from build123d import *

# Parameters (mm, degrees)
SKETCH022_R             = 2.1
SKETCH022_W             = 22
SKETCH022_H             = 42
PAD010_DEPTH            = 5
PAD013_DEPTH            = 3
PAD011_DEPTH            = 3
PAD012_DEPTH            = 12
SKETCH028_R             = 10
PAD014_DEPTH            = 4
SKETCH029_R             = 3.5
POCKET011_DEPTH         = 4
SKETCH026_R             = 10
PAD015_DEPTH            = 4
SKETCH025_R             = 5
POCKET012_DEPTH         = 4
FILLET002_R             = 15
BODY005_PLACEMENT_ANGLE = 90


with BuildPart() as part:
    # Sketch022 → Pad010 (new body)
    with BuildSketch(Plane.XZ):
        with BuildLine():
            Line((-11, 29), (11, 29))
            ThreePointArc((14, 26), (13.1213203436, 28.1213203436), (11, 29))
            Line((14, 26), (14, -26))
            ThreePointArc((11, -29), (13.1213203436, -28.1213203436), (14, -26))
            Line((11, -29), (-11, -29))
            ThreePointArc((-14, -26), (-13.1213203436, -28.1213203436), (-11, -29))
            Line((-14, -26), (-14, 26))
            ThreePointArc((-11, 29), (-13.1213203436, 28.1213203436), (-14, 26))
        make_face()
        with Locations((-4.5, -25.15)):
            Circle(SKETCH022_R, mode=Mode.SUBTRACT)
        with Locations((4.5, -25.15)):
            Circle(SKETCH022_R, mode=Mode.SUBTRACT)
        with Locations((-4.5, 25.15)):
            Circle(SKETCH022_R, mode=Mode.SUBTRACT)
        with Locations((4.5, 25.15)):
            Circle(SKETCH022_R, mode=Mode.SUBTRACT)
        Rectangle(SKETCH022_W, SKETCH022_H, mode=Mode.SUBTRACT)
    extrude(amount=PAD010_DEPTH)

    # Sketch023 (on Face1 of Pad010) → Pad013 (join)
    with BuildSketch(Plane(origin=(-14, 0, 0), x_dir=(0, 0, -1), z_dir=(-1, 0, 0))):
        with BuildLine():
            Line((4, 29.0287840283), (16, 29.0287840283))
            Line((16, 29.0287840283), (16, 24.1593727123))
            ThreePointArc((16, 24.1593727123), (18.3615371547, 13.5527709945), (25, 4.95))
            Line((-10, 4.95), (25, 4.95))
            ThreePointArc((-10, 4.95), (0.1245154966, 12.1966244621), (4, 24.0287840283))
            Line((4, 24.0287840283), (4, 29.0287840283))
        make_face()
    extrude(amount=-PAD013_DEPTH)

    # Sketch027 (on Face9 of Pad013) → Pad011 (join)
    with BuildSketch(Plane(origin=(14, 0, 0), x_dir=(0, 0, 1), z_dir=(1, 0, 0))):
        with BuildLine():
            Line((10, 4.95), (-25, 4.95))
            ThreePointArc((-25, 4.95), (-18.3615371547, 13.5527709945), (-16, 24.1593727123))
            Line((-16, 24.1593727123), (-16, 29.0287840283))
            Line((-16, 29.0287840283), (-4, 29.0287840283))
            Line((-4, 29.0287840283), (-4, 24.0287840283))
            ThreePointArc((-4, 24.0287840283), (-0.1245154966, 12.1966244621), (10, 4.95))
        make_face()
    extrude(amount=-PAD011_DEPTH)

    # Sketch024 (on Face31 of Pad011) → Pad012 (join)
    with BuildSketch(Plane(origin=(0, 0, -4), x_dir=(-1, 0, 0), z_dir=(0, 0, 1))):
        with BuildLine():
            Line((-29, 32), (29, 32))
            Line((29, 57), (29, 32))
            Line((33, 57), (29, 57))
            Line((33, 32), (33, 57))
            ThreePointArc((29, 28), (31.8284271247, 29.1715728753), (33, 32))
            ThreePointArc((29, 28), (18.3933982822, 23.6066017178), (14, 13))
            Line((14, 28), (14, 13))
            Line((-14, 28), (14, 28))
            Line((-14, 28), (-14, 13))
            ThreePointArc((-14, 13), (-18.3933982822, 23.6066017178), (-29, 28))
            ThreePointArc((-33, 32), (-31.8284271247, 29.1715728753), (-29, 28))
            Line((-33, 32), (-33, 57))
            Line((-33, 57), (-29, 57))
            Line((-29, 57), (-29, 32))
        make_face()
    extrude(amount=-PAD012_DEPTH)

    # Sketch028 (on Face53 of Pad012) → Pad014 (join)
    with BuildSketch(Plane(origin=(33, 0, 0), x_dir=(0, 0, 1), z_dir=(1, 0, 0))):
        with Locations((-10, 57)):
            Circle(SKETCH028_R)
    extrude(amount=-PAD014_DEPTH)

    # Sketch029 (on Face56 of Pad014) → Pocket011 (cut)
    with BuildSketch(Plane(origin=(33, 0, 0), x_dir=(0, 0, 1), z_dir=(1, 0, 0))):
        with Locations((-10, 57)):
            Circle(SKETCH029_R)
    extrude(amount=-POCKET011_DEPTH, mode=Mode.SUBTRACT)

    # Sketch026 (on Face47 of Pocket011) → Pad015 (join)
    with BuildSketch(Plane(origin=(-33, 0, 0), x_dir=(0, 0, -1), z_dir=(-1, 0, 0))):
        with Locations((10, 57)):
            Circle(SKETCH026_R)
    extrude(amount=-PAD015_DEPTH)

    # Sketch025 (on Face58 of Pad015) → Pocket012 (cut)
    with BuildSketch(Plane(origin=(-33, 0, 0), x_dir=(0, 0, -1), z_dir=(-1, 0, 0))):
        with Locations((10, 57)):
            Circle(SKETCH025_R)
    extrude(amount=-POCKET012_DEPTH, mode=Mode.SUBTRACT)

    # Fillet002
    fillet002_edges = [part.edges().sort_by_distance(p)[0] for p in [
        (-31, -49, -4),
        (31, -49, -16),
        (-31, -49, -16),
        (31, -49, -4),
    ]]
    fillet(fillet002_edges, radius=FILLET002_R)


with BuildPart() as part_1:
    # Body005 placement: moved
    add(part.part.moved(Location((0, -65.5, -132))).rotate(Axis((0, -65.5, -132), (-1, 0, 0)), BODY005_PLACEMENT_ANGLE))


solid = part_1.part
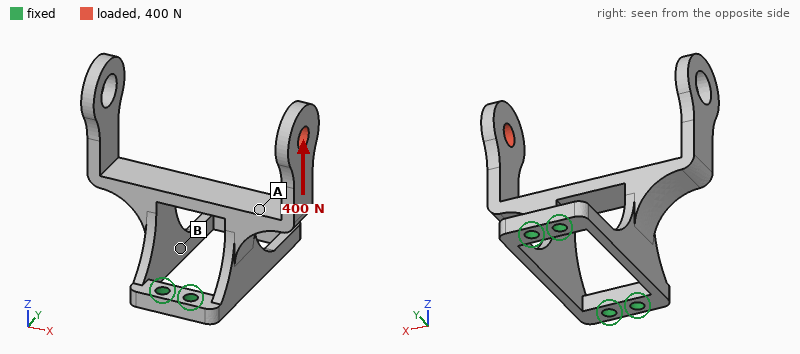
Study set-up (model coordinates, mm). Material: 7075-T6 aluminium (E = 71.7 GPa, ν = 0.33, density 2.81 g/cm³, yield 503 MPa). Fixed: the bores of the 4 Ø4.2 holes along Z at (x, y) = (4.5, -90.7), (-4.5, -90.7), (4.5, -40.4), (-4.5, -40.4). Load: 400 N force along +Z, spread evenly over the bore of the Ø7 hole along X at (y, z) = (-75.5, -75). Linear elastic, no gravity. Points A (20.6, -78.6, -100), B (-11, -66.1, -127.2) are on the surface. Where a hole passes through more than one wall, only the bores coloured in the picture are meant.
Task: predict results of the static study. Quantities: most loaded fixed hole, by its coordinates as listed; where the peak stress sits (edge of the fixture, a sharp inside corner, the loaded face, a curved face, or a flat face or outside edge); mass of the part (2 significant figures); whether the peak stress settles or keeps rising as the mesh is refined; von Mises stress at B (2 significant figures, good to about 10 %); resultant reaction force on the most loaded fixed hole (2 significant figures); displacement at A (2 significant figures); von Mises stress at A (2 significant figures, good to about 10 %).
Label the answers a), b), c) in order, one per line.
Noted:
a) (4.5, -90.7)
b) edge of the fixture
c) 38 g
d) keeps rising
e) 13 MPa
f) 560 N
g) 0.20 mm
h) 54 MPa
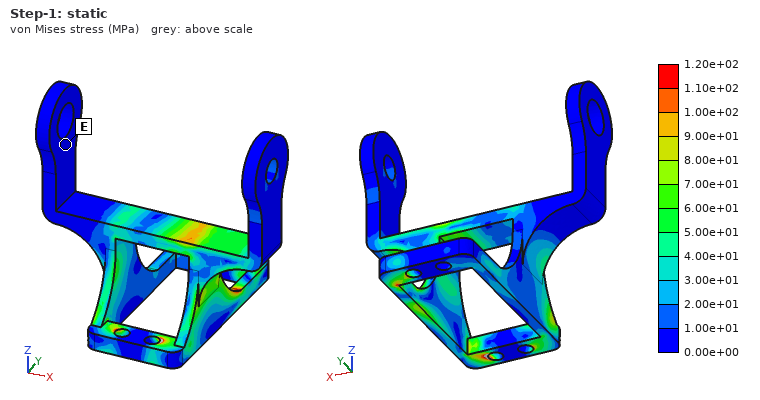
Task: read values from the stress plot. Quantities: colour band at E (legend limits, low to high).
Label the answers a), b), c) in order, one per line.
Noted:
a) 0.00e+00 to 1.00e+01 MPa
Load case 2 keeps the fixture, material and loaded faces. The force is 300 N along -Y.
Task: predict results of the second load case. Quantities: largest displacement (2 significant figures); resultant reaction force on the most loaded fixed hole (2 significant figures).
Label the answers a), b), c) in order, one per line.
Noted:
a) 1.0 mm
b) 460 N
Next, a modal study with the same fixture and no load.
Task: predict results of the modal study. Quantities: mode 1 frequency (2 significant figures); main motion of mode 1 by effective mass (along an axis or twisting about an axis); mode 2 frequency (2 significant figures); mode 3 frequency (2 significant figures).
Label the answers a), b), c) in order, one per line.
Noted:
a) 910 Hz
b) along X
c) 1400 Hz
d) 1500 Hz
